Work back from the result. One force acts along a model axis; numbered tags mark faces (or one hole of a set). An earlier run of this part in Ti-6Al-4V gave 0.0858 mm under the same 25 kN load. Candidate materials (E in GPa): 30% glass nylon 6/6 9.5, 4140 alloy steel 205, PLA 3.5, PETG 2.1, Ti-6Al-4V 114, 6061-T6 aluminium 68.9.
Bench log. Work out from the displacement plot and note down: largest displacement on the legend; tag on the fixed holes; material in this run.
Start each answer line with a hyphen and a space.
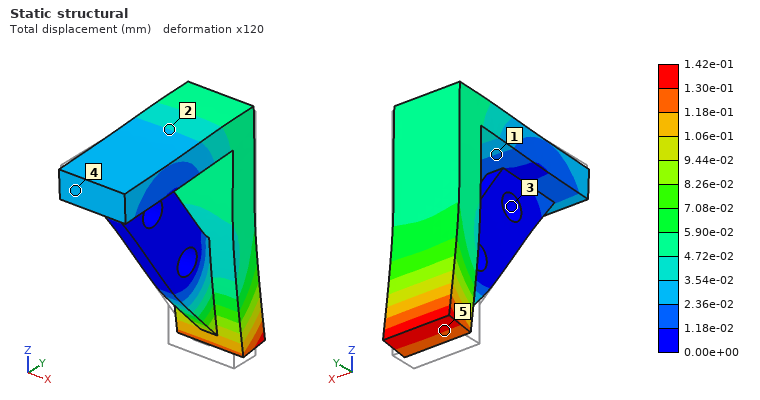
- 1.42e-01 mm
- 3
- 6061-T6 aluminium
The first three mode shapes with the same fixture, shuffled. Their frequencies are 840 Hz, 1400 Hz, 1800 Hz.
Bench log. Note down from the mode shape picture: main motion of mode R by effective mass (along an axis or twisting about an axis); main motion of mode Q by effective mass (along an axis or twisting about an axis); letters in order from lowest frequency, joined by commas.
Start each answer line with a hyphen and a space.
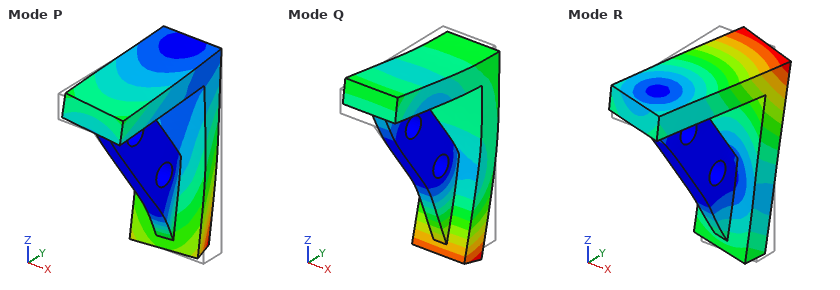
- along X
- along Z
- R, P, Q
